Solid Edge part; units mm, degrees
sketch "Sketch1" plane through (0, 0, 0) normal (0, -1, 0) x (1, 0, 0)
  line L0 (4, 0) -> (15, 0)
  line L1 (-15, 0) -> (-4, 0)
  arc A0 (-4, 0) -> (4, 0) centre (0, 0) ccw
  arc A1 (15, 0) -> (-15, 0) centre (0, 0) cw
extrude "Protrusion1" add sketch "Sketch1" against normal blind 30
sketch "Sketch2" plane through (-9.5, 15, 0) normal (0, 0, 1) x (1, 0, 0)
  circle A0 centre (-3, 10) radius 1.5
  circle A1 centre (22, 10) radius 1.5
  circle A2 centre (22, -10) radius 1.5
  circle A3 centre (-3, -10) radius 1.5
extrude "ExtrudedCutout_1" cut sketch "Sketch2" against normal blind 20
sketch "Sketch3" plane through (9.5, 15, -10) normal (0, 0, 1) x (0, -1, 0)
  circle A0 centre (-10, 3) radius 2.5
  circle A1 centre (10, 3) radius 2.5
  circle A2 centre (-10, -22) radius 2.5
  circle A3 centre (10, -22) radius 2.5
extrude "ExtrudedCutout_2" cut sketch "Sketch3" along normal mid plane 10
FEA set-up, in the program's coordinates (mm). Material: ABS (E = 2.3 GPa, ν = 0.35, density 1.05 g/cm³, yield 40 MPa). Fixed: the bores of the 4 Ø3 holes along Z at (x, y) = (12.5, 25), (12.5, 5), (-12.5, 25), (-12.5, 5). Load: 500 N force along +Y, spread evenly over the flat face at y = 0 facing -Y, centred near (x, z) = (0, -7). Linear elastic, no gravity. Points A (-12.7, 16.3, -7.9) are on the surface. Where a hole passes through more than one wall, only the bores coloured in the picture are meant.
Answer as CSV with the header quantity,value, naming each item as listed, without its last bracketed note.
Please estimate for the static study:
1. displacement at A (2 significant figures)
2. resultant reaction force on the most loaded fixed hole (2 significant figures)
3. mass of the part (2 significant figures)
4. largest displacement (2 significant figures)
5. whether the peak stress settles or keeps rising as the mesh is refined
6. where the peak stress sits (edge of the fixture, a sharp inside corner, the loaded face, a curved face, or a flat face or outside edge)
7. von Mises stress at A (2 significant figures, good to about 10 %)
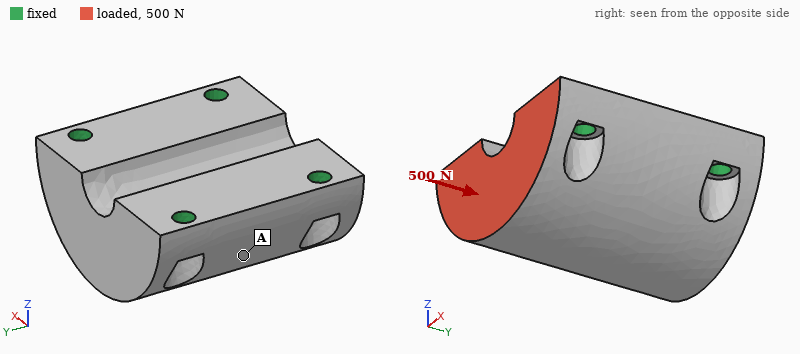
quantity,value
displacement at A,8.7 µm
resultant reaction force on the most loaded fixed hole,170 N
mass of the part,9.9 g
largest displacement,32 µm
whether the peak stress settles or keeps rising as the mesh is refined,keeps rising
where the peak stress sits,edge of the fixture
von Mises stress at A,1.5 MPa
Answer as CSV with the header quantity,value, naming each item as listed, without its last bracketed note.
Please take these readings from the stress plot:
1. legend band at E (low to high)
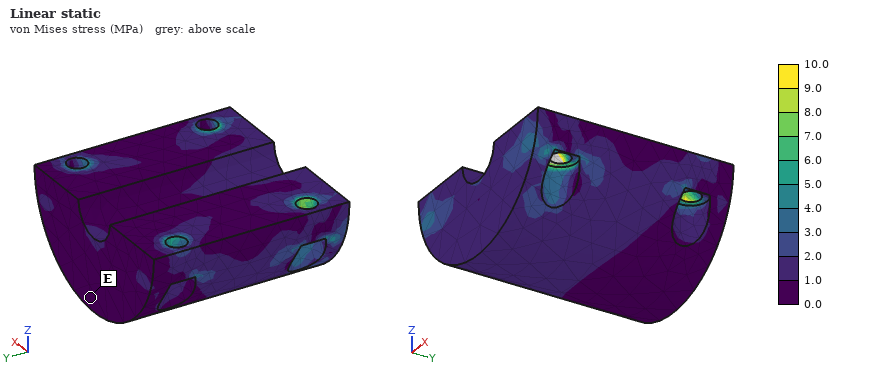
quantity,value
legend band at E,0.0 to 1.0 MPa
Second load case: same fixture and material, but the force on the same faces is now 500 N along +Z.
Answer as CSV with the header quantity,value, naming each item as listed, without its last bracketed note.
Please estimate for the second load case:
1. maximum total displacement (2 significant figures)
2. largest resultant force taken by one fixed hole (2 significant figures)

quantity,value
maximum total displacement,74 µm
largest resultant force taken by one fixed hole,310 N
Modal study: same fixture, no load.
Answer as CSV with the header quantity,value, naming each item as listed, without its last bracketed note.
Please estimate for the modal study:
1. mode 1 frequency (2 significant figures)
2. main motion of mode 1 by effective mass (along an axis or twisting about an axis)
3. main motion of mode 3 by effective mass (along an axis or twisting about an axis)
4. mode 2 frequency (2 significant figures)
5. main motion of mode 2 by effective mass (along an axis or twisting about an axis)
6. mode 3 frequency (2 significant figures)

quantity,value
mode 1 frequency,8600 Hz
main motion of mode 1 by effective mass,along Y
main motion of mode 3 by effective mass,along X
mode 2 frequency,9500 Hz
main motion of mode 2 by effective mass,along Z
mode 3 frequency,11 kHz
